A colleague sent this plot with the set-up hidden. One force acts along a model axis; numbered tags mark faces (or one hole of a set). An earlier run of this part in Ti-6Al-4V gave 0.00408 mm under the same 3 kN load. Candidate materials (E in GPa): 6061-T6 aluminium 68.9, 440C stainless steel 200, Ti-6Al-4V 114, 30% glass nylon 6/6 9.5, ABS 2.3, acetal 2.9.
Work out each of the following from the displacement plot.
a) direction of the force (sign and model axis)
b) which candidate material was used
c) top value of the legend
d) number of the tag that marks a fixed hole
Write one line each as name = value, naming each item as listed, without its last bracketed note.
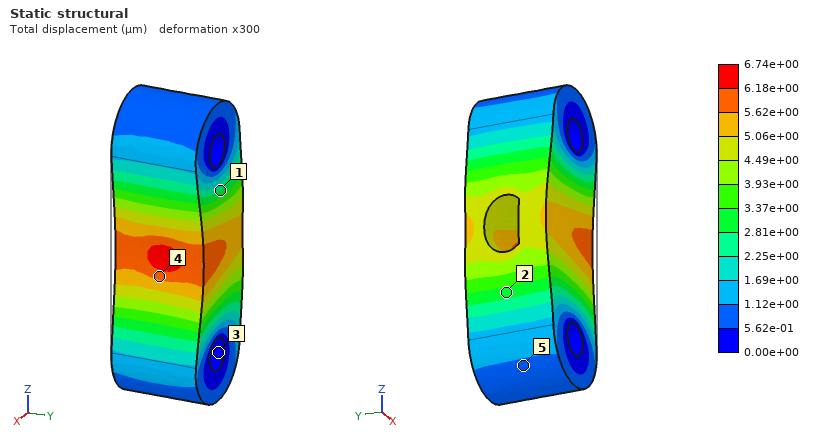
direction of the force = -X
which candidate material was used = 6061-T6 aluminium
top value of the legend = 6.74e+00 µm
number of the tag that marks a fixed hole = 3
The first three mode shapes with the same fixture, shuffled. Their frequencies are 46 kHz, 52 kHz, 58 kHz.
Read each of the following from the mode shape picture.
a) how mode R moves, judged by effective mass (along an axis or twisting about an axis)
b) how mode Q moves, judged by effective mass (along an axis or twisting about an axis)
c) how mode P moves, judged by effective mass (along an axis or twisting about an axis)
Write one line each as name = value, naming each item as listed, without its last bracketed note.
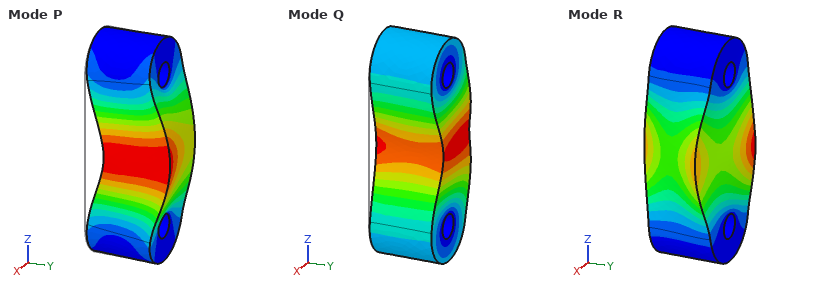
how mode R moves, judged by effective mass = twisting about Z
how mode Q moves, judged by effective mass = along X
how mode P moves, judged by effective mass = along Y
